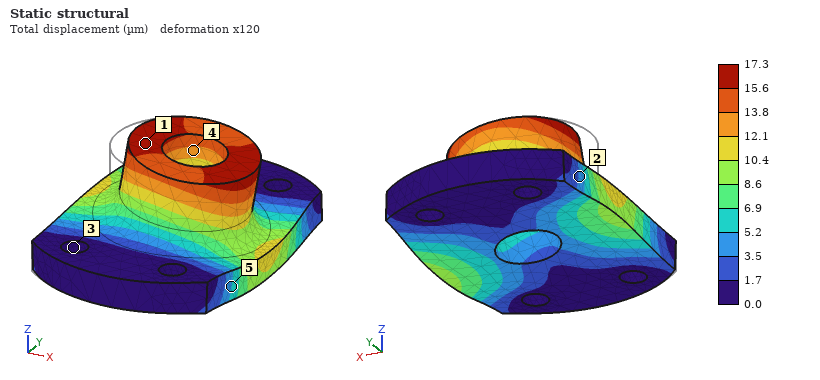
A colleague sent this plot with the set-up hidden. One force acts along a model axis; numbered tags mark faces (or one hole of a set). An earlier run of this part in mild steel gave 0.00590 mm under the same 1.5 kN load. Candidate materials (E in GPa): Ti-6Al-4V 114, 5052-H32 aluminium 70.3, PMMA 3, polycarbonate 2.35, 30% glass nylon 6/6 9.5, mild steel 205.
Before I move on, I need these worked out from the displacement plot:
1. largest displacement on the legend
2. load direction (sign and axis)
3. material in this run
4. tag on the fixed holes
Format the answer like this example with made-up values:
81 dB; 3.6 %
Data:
17.3 µm; +X; 5052-H32 aluminium; 3
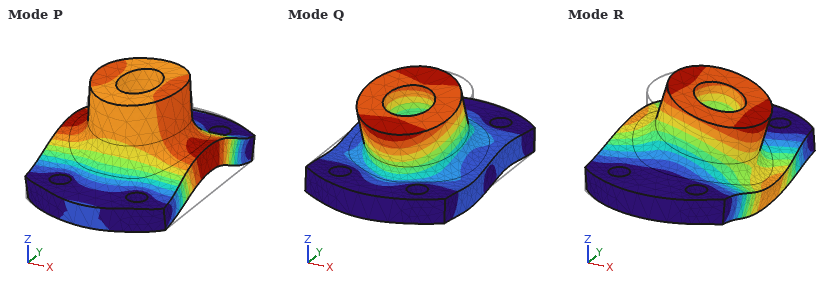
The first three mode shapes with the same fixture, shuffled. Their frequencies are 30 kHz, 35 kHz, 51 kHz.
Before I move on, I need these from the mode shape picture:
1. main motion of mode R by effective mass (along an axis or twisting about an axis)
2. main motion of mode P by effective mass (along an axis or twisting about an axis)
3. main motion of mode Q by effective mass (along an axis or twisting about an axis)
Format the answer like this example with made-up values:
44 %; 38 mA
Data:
along X; along Z; along Y
